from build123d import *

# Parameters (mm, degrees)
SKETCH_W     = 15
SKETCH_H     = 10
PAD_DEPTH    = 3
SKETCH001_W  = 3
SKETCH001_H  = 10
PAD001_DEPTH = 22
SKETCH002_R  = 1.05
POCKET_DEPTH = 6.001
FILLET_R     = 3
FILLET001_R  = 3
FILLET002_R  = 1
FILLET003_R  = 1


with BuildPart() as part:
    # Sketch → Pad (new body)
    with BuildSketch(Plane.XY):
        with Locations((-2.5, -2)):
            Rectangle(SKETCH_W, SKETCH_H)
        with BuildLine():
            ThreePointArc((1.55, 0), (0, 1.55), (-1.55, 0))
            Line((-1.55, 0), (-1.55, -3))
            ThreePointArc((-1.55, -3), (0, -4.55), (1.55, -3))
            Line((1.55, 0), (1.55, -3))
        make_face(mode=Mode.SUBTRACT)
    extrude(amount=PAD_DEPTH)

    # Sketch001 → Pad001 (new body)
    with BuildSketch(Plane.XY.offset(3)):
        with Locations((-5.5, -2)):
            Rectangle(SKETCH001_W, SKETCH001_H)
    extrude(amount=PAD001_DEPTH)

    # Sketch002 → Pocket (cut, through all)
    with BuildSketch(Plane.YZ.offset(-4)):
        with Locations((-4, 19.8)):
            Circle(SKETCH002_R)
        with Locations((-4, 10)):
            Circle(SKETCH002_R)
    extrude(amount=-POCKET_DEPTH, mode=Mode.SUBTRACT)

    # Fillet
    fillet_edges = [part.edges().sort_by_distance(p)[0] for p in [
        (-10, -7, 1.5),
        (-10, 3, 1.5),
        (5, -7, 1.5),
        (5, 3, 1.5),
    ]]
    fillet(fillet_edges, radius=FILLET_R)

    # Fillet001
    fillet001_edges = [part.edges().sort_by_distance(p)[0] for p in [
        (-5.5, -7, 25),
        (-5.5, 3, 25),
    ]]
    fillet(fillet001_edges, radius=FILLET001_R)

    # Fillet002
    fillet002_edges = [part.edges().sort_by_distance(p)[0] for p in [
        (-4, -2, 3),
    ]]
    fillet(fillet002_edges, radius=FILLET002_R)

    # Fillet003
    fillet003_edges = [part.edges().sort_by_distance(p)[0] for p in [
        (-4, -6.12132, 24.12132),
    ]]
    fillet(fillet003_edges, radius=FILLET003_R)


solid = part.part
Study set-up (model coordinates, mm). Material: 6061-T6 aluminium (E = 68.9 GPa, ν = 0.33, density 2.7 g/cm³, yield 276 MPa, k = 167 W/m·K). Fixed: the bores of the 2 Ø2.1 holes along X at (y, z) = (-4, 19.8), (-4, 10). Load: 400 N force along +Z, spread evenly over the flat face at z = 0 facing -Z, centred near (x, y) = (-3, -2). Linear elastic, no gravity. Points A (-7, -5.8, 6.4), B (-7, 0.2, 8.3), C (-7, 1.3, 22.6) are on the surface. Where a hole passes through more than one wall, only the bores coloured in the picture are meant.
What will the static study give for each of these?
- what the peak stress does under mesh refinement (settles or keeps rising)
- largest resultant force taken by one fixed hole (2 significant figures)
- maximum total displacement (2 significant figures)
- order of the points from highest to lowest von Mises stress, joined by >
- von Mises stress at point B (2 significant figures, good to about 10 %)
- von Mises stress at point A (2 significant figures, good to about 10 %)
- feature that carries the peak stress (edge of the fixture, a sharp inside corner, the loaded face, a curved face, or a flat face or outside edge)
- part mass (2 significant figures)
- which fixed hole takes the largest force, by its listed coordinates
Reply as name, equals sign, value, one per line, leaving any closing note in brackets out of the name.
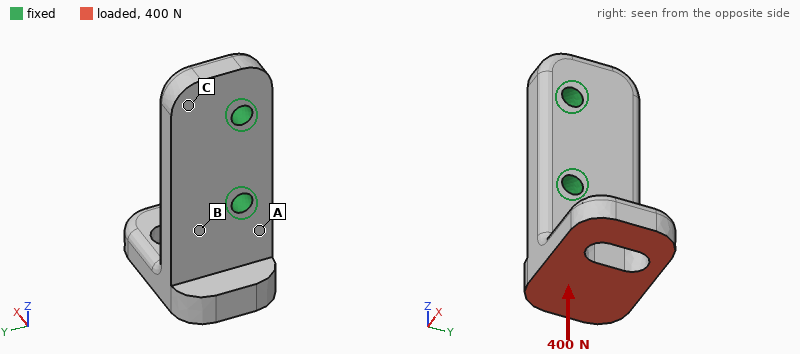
what the peak stress does under mesh refinement = keeps rising
largest resultant force taken by one fixed hole = 330 N
maximum total displacement = 99 µm
order of the points from highest to lowest von Mises stress, joined by > = A > B > C
von Mises stress at point B = 43 MPa
von Mises stress at point A = 66 MPa
feature that carries the peak stress = edge of the fixture
part mass = 2.7 g
which fixed hole takes the largest force, by its listed coordinates = (-4, 10)
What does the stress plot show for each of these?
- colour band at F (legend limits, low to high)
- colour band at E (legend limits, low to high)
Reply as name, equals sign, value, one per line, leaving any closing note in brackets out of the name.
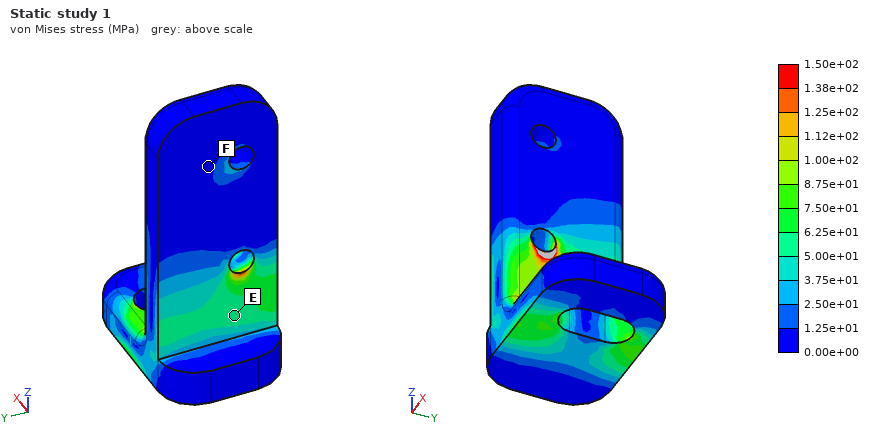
colour band at F = 0.00e+00 to 1.25e+01 MPa
colour band at E = 5.00e+01 to 6.25e+01 MPa
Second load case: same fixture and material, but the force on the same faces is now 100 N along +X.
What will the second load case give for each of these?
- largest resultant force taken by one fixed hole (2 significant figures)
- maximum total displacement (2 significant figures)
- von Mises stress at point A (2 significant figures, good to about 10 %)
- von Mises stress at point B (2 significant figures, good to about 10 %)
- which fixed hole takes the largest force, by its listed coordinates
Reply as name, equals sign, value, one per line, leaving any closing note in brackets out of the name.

largest resultant force taken by one fixed hole = 130 N
maximum total displacement = 46 µm
von Mises stress at point A = 47 MPa
von Mises stress at point B = 38 MPa
which fixed hole takes the largest force, by its listed coordinates = (-4, 10)
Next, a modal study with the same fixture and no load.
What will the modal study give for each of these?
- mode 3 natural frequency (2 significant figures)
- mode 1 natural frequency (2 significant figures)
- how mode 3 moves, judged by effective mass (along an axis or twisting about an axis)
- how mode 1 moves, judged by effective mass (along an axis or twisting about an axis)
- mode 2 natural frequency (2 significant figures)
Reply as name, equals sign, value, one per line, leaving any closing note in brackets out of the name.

mode 3 natural frequency = 23 kHz
mode 1 natural frequency = 9000 Hz
how mode 3 moves, judged by effective mass = along X
how mode 1 moves, judged by effective mass = along X
mode 2 natural frequency = 13 kHz
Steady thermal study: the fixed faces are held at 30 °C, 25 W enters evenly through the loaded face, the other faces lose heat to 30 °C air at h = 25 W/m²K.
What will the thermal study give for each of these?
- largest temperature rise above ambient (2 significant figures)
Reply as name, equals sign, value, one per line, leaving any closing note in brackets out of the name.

largest temperature rise above ambient = 68 K
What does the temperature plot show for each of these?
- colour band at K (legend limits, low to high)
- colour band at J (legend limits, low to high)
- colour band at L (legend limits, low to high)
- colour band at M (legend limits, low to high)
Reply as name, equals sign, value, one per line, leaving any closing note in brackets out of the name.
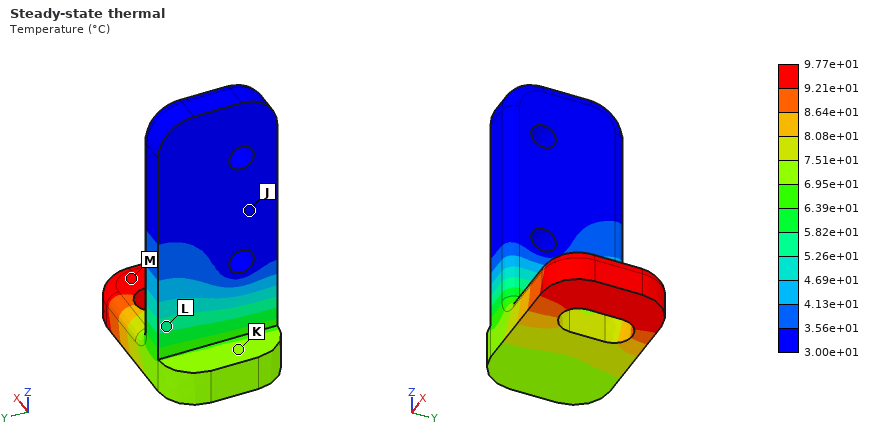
colour band at K = 6.95e+01 to 7.51e+01 °C
colour band at J = 3.00e+01 to 3.56e+01 °C
colour band at L = 5.26e+01 to 5.82e+01 °C
colour band at M = 9.21e+01 to 9.77e+01 °C
